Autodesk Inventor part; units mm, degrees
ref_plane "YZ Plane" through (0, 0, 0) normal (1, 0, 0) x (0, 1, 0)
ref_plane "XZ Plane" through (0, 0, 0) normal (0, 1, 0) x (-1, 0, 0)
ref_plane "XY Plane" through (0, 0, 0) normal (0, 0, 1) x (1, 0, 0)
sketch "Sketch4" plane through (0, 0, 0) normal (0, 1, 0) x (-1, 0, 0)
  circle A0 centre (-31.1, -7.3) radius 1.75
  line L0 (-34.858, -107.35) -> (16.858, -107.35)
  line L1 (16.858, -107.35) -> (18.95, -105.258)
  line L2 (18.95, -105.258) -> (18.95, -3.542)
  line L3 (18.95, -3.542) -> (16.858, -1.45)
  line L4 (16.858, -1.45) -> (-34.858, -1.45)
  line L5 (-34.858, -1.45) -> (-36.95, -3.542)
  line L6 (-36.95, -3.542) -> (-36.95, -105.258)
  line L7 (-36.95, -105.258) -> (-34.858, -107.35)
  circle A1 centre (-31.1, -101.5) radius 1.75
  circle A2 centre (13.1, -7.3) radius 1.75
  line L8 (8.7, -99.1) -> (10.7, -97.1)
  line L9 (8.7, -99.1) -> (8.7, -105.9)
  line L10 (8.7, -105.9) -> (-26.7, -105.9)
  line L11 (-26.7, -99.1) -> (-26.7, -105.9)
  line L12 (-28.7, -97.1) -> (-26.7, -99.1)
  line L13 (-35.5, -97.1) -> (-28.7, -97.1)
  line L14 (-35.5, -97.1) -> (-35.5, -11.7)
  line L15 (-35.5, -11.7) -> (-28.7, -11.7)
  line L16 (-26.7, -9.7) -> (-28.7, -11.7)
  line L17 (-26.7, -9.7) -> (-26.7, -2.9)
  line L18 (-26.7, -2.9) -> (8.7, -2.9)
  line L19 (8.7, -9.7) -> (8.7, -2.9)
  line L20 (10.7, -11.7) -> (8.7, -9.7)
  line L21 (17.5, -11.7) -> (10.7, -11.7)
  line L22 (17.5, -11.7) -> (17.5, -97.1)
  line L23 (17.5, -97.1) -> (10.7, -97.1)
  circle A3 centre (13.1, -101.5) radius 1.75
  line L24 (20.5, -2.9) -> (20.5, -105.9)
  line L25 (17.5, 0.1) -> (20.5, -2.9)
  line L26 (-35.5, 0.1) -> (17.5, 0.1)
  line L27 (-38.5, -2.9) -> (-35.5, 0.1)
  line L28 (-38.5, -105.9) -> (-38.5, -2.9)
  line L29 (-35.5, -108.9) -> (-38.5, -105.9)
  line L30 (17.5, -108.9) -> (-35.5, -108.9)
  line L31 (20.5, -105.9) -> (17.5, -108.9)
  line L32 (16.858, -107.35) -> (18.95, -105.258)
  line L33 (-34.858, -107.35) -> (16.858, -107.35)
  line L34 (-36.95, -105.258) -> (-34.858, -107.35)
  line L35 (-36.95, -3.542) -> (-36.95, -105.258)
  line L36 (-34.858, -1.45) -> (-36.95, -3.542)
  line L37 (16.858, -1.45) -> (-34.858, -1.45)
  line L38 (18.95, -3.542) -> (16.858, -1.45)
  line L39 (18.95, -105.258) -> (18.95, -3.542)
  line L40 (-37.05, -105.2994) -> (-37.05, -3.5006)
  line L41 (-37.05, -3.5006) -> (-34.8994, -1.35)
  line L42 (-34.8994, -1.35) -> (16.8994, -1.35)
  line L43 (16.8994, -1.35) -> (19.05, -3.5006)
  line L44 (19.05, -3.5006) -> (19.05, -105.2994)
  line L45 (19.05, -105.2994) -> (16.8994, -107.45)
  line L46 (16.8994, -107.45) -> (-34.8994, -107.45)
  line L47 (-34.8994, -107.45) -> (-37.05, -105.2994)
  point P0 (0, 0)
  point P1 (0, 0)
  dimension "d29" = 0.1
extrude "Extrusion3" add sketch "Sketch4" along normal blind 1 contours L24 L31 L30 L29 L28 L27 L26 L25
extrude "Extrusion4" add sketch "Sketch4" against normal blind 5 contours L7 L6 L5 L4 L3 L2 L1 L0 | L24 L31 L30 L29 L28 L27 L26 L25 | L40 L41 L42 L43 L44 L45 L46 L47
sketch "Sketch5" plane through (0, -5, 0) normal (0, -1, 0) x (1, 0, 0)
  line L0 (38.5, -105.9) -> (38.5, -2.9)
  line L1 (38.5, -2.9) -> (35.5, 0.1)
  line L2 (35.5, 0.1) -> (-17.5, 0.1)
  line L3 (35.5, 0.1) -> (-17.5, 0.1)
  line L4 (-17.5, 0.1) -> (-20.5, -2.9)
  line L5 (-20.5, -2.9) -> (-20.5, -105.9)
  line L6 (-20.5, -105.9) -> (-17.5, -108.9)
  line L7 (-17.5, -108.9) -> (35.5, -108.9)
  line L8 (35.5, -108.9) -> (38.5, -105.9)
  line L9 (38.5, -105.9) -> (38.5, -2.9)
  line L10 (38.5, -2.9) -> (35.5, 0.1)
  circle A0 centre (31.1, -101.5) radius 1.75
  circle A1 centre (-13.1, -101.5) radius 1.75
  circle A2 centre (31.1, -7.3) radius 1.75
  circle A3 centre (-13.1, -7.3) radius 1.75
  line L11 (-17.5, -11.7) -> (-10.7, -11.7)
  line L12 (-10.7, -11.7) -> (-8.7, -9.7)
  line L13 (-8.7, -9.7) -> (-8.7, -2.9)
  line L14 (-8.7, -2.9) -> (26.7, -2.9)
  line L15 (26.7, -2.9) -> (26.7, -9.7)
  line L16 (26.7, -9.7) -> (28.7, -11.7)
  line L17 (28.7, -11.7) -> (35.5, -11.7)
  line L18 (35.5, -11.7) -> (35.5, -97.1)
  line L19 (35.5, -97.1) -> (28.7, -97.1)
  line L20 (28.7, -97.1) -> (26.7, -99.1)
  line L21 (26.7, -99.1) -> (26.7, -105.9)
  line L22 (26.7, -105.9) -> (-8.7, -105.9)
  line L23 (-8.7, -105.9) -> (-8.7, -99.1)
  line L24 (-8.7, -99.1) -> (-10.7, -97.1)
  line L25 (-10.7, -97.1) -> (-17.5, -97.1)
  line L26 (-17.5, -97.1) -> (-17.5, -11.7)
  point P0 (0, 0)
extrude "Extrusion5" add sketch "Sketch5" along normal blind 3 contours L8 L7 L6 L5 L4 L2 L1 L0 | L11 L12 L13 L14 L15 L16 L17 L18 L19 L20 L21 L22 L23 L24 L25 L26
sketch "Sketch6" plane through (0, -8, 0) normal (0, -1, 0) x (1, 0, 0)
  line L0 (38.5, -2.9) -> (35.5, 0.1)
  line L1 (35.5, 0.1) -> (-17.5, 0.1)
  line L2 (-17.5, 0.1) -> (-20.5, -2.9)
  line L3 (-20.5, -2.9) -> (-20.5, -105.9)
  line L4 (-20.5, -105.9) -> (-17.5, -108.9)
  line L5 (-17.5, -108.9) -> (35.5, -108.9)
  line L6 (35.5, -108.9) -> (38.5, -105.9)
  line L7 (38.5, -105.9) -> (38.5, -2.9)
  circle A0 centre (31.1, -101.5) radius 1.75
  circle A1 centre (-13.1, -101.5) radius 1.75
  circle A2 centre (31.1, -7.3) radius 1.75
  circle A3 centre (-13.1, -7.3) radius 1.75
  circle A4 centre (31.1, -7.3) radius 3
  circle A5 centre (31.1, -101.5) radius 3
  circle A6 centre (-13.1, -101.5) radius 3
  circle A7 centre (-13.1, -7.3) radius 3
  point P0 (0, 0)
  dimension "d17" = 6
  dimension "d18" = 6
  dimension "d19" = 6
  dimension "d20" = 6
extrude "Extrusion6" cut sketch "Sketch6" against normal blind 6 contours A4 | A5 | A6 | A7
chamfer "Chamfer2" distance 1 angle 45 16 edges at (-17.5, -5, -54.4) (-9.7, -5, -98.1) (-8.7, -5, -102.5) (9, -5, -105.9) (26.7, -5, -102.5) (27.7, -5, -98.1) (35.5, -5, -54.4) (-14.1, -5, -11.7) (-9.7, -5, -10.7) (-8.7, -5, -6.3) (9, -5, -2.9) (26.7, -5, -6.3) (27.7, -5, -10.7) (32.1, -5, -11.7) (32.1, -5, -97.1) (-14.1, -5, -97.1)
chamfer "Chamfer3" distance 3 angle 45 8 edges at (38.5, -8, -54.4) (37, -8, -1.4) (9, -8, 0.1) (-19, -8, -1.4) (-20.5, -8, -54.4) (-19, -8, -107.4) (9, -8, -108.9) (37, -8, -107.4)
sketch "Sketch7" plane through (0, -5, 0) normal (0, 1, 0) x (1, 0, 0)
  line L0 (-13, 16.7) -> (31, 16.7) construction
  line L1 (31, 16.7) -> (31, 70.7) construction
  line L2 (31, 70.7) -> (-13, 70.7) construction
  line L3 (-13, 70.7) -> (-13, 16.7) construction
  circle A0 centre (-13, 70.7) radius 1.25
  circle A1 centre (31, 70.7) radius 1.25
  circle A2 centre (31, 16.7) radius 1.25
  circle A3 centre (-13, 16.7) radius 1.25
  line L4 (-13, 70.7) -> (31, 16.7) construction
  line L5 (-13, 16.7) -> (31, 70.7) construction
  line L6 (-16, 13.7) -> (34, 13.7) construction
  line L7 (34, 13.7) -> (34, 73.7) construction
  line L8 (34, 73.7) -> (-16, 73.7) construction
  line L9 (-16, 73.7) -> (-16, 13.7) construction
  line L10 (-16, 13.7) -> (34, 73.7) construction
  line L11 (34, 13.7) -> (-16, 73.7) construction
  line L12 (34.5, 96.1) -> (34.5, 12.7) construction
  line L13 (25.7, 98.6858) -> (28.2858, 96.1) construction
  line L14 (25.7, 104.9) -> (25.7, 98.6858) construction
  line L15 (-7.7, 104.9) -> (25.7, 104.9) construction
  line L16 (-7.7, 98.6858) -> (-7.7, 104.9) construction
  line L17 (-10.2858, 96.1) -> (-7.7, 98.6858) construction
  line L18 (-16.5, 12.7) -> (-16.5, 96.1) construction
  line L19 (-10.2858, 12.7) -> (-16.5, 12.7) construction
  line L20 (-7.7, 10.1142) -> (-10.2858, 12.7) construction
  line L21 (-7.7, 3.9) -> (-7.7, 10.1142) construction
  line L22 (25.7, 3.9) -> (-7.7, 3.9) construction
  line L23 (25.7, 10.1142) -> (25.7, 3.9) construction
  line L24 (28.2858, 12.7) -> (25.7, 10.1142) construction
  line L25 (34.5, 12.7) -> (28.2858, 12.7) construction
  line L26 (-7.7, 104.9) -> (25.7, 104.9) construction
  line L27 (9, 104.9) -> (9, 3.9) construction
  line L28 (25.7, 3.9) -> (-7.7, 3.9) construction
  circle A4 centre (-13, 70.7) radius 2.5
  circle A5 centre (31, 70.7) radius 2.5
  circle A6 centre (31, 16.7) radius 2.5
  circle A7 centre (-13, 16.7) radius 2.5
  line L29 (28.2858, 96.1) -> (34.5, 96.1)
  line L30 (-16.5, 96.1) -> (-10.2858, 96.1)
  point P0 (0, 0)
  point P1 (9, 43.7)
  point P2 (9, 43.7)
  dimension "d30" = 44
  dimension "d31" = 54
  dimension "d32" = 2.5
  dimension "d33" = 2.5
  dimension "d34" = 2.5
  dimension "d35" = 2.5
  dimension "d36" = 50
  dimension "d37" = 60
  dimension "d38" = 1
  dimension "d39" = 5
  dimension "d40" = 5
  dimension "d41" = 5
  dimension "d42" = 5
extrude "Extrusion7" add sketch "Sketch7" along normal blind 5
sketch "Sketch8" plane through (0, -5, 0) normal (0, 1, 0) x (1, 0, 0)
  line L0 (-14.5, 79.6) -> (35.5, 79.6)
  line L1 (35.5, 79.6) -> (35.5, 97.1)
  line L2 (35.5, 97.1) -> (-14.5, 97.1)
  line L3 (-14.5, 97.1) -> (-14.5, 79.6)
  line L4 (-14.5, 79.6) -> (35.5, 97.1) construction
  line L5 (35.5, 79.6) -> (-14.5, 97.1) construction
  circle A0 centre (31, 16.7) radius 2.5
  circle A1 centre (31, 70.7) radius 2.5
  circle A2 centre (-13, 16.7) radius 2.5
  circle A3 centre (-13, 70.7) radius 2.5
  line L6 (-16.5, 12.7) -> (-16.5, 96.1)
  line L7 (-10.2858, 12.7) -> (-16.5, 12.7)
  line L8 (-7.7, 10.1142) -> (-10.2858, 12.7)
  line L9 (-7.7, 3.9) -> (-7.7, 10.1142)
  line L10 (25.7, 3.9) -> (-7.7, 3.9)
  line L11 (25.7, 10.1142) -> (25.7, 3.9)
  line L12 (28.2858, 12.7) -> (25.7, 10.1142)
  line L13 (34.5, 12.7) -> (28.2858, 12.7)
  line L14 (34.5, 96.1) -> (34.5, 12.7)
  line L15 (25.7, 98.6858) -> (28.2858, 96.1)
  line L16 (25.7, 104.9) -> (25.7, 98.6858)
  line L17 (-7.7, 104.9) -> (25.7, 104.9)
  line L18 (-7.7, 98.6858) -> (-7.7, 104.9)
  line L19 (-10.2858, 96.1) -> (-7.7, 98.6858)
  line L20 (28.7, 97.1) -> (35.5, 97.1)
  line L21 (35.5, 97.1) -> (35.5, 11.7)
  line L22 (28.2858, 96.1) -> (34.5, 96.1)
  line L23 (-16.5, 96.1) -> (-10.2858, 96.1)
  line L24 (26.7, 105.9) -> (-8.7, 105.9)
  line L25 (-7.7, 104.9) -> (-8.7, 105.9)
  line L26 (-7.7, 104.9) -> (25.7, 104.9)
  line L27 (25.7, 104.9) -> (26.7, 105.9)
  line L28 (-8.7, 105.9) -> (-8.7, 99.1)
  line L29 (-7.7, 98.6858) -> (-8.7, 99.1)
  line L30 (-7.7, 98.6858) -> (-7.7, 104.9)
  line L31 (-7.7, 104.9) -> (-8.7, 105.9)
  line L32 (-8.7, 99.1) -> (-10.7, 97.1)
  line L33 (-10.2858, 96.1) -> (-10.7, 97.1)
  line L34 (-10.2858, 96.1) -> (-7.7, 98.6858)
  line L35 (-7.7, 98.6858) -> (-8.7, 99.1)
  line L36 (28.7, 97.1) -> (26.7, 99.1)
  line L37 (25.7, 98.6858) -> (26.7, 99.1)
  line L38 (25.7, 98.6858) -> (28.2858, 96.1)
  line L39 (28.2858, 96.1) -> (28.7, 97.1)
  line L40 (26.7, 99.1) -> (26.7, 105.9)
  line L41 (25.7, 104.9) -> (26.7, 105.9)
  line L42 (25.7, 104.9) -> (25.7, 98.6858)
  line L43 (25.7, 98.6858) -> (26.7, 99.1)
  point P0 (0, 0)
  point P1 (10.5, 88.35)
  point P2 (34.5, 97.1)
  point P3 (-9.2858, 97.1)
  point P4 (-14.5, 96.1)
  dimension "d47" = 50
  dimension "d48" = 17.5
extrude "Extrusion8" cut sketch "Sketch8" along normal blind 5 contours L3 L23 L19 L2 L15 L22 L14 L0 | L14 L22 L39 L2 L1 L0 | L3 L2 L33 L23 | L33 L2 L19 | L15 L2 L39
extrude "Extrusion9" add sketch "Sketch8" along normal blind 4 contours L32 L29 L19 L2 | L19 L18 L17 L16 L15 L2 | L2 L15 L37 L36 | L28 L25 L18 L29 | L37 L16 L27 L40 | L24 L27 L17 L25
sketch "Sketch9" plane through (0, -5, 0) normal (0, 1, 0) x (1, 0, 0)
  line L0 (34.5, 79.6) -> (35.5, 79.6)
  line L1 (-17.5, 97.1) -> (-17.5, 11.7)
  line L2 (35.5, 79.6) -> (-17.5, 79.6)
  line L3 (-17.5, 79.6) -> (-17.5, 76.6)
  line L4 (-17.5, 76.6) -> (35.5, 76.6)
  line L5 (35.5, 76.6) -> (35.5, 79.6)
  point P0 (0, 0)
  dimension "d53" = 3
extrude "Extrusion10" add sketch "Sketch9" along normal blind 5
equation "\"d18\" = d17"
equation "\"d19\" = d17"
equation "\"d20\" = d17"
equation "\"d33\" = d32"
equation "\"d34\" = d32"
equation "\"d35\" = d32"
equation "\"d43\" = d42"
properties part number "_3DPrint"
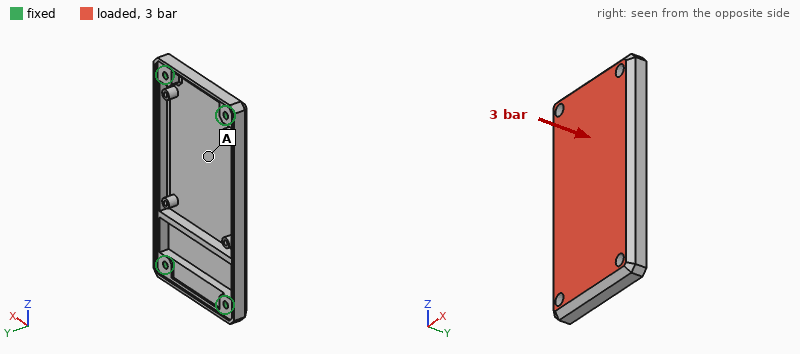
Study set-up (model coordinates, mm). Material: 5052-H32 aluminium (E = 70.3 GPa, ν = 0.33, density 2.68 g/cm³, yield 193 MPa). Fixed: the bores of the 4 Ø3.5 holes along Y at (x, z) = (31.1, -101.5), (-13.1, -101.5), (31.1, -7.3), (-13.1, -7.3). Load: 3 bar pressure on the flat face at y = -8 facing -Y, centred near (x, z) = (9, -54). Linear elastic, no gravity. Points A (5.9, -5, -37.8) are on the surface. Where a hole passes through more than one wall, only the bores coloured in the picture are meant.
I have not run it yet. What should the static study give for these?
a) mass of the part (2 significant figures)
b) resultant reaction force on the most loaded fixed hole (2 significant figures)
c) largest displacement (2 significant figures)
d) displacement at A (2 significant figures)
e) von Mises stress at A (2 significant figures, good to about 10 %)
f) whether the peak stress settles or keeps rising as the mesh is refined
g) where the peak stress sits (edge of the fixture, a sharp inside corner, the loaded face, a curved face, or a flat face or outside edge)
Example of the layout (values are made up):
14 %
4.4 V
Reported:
70 g
830 N
0.16 mm
0.14 mm
25 MPa
keeps rising
edge of the fixture
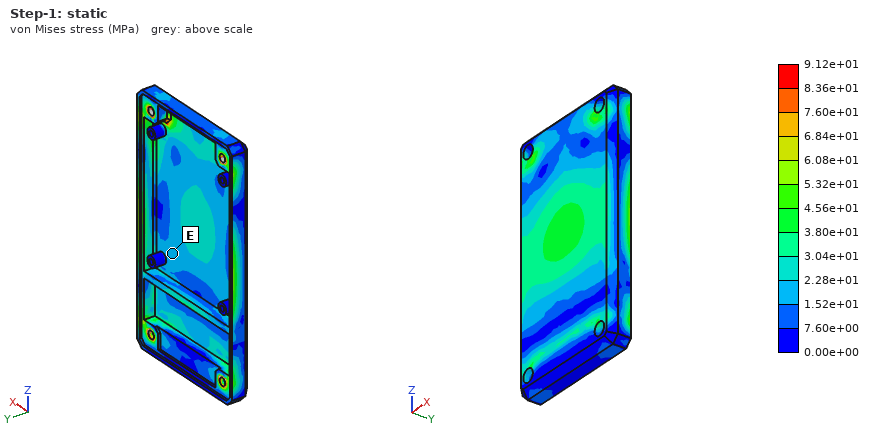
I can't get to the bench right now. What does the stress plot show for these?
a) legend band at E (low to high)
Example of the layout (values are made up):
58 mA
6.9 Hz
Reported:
1.52e+01 to 2.28e+01 MPa
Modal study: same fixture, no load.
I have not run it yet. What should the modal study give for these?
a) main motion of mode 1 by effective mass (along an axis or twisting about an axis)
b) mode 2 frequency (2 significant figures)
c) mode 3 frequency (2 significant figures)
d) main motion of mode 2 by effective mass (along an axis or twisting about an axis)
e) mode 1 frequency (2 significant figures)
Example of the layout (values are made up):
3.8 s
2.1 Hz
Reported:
along Y
3700 Hz
5400 Hz
twisting about Z
2600 Hz
